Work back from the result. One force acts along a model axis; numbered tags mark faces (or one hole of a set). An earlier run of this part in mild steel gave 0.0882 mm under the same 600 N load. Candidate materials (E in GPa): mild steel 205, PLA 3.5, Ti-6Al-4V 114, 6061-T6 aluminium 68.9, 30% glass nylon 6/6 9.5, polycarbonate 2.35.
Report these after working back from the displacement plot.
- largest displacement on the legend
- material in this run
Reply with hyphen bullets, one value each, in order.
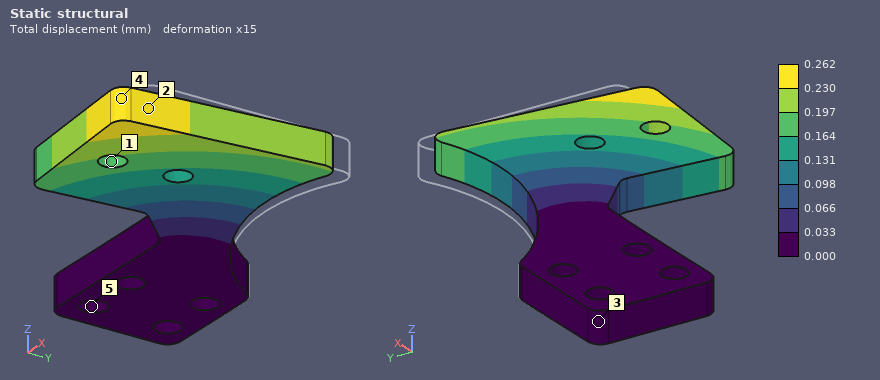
- 0.262 mm
- 6061-T6 aluminium
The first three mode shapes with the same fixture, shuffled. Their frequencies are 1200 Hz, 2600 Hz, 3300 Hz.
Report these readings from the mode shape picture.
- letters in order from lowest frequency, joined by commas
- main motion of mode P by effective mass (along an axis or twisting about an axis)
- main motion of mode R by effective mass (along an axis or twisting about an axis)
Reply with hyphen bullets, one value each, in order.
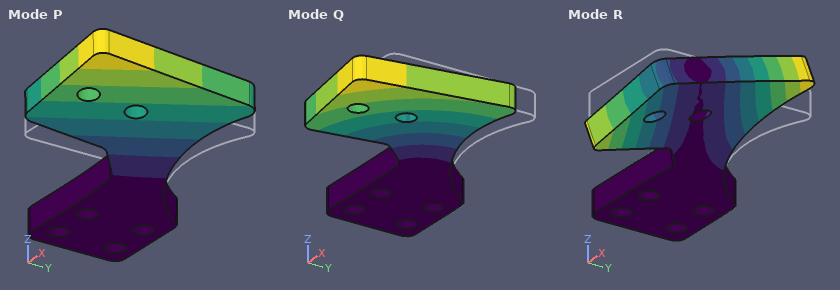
- P, Q, R
- along Z
- twisting about X
